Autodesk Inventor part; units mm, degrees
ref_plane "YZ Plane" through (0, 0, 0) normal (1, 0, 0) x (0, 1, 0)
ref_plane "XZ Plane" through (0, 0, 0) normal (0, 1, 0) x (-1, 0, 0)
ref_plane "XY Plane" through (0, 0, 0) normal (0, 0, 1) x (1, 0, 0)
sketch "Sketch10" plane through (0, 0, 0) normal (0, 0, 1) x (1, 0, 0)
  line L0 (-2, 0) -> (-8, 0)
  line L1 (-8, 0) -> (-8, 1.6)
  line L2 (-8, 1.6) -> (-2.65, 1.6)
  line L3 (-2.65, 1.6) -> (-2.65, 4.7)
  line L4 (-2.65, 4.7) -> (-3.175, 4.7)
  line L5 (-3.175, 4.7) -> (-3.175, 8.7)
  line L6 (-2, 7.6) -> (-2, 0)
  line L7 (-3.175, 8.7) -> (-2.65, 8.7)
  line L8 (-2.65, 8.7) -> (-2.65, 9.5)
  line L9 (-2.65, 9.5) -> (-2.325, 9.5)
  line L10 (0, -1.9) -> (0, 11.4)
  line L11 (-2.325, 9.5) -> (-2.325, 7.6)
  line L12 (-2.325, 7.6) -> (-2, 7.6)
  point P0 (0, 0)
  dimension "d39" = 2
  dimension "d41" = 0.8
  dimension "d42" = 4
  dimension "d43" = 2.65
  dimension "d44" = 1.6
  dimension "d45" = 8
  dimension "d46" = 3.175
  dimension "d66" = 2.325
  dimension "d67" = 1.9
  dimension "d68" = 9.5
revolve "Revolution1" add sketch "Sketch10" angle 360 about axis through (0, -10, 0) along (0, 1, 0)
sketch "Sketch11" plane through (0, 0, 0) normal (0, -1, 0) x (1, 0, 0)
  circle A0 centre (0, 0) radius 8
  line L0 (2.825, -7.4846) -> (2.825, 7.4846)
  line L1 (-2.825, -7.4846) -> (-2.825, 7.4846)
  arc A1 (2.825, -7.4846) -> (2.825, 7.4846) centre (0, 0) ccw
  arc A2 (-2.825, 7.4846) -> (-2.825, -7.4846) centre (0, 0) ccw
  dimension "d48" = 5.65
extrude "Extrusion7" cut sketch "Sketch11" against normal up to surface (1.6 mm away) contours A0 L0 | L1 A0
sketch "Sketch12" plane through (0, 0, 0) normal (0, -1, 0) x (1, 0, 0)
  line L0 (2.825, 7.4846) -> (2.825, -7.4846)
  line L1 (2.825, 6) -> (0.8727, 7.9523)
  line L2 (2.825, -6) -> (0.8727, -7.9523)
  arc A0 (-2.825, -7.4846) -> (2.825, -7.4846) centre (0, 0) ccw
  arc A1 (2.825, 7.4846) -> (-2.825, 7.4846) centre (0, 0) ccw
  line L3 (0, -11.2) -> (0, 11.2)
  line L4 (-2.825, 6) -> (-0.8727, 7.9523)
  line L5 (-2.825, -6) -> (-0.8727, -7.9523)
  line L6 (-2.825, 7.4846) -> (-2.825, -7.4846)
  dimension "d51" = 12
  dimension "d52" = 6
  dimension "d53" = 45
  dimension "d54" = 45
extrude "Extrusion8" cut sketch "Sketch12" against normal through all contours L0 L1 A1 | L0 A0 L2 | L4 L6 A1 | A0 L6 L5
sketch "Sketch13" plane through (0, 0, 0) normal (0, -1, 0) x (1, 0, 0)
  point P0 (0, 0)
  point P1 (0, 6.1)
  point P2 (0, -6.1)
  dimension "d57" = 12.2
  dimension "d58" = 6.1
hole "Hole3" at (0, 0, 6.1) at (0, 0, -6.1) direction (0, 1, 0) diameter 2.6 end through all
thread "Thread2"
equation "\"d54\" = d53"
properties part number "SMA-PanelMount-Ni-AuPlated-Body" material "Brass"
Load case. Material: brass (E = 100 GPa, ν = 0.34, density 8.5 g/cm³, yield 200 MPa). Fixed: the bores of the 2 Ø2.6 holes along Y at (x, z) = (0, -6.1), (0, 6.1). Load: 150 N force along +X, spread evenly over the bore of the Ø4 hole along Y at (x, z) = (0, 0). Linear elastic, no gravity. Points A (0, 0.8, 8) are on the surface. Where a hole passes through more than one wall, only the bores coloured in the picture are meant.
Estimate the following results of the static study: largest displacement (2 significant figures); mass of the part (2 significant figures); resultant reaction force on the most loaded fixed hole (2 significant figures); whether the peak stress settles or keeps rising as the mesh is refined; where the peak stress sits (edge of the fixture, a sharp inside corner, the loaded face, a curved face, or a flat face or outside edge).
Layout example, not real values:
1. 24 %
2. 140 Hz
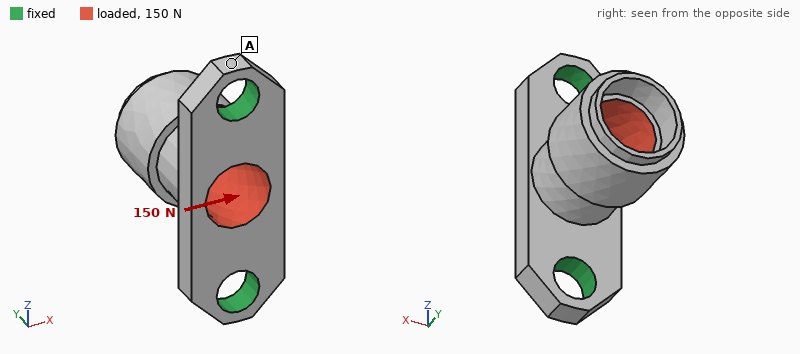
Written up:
1. 30 µm
2. 1.7 g
3. 75 N
4. keeps rising
5. edge of the fixture
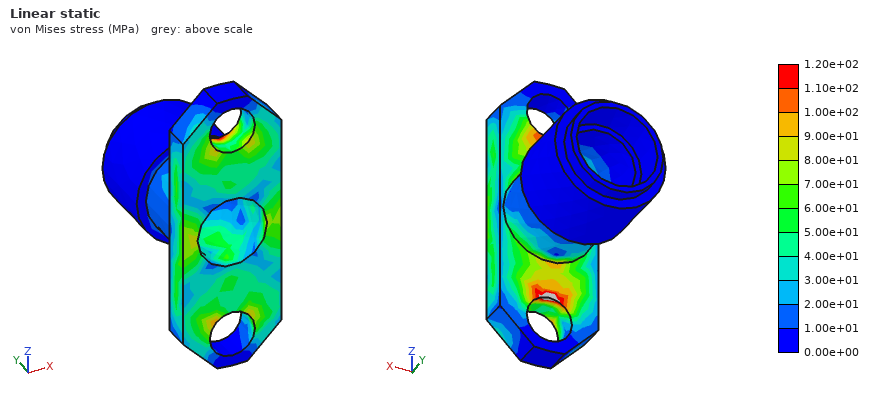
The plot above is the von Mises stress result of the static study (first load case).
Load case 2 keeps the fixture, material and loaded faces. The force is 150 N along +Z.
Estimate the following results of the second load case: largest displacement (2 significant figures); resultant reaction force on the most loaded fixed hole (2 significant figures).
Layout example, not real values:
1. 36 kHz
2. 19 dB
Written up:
1. 9.0 µm
2. 96 N
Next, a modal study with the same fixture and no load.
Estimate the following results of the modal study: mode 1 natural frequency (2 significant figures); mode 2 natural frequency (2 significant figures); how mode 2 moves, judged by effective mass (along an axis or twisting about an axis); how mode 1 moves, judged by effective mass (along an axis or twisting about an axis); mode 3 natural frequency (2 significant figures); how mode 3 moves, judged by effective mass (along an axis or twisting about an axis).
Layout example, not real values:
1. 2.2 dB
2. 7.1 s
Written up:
1. 11 kHz
2. 19 kHz
3. along Z
4. along X
5. 30 kHz
6. along Y
